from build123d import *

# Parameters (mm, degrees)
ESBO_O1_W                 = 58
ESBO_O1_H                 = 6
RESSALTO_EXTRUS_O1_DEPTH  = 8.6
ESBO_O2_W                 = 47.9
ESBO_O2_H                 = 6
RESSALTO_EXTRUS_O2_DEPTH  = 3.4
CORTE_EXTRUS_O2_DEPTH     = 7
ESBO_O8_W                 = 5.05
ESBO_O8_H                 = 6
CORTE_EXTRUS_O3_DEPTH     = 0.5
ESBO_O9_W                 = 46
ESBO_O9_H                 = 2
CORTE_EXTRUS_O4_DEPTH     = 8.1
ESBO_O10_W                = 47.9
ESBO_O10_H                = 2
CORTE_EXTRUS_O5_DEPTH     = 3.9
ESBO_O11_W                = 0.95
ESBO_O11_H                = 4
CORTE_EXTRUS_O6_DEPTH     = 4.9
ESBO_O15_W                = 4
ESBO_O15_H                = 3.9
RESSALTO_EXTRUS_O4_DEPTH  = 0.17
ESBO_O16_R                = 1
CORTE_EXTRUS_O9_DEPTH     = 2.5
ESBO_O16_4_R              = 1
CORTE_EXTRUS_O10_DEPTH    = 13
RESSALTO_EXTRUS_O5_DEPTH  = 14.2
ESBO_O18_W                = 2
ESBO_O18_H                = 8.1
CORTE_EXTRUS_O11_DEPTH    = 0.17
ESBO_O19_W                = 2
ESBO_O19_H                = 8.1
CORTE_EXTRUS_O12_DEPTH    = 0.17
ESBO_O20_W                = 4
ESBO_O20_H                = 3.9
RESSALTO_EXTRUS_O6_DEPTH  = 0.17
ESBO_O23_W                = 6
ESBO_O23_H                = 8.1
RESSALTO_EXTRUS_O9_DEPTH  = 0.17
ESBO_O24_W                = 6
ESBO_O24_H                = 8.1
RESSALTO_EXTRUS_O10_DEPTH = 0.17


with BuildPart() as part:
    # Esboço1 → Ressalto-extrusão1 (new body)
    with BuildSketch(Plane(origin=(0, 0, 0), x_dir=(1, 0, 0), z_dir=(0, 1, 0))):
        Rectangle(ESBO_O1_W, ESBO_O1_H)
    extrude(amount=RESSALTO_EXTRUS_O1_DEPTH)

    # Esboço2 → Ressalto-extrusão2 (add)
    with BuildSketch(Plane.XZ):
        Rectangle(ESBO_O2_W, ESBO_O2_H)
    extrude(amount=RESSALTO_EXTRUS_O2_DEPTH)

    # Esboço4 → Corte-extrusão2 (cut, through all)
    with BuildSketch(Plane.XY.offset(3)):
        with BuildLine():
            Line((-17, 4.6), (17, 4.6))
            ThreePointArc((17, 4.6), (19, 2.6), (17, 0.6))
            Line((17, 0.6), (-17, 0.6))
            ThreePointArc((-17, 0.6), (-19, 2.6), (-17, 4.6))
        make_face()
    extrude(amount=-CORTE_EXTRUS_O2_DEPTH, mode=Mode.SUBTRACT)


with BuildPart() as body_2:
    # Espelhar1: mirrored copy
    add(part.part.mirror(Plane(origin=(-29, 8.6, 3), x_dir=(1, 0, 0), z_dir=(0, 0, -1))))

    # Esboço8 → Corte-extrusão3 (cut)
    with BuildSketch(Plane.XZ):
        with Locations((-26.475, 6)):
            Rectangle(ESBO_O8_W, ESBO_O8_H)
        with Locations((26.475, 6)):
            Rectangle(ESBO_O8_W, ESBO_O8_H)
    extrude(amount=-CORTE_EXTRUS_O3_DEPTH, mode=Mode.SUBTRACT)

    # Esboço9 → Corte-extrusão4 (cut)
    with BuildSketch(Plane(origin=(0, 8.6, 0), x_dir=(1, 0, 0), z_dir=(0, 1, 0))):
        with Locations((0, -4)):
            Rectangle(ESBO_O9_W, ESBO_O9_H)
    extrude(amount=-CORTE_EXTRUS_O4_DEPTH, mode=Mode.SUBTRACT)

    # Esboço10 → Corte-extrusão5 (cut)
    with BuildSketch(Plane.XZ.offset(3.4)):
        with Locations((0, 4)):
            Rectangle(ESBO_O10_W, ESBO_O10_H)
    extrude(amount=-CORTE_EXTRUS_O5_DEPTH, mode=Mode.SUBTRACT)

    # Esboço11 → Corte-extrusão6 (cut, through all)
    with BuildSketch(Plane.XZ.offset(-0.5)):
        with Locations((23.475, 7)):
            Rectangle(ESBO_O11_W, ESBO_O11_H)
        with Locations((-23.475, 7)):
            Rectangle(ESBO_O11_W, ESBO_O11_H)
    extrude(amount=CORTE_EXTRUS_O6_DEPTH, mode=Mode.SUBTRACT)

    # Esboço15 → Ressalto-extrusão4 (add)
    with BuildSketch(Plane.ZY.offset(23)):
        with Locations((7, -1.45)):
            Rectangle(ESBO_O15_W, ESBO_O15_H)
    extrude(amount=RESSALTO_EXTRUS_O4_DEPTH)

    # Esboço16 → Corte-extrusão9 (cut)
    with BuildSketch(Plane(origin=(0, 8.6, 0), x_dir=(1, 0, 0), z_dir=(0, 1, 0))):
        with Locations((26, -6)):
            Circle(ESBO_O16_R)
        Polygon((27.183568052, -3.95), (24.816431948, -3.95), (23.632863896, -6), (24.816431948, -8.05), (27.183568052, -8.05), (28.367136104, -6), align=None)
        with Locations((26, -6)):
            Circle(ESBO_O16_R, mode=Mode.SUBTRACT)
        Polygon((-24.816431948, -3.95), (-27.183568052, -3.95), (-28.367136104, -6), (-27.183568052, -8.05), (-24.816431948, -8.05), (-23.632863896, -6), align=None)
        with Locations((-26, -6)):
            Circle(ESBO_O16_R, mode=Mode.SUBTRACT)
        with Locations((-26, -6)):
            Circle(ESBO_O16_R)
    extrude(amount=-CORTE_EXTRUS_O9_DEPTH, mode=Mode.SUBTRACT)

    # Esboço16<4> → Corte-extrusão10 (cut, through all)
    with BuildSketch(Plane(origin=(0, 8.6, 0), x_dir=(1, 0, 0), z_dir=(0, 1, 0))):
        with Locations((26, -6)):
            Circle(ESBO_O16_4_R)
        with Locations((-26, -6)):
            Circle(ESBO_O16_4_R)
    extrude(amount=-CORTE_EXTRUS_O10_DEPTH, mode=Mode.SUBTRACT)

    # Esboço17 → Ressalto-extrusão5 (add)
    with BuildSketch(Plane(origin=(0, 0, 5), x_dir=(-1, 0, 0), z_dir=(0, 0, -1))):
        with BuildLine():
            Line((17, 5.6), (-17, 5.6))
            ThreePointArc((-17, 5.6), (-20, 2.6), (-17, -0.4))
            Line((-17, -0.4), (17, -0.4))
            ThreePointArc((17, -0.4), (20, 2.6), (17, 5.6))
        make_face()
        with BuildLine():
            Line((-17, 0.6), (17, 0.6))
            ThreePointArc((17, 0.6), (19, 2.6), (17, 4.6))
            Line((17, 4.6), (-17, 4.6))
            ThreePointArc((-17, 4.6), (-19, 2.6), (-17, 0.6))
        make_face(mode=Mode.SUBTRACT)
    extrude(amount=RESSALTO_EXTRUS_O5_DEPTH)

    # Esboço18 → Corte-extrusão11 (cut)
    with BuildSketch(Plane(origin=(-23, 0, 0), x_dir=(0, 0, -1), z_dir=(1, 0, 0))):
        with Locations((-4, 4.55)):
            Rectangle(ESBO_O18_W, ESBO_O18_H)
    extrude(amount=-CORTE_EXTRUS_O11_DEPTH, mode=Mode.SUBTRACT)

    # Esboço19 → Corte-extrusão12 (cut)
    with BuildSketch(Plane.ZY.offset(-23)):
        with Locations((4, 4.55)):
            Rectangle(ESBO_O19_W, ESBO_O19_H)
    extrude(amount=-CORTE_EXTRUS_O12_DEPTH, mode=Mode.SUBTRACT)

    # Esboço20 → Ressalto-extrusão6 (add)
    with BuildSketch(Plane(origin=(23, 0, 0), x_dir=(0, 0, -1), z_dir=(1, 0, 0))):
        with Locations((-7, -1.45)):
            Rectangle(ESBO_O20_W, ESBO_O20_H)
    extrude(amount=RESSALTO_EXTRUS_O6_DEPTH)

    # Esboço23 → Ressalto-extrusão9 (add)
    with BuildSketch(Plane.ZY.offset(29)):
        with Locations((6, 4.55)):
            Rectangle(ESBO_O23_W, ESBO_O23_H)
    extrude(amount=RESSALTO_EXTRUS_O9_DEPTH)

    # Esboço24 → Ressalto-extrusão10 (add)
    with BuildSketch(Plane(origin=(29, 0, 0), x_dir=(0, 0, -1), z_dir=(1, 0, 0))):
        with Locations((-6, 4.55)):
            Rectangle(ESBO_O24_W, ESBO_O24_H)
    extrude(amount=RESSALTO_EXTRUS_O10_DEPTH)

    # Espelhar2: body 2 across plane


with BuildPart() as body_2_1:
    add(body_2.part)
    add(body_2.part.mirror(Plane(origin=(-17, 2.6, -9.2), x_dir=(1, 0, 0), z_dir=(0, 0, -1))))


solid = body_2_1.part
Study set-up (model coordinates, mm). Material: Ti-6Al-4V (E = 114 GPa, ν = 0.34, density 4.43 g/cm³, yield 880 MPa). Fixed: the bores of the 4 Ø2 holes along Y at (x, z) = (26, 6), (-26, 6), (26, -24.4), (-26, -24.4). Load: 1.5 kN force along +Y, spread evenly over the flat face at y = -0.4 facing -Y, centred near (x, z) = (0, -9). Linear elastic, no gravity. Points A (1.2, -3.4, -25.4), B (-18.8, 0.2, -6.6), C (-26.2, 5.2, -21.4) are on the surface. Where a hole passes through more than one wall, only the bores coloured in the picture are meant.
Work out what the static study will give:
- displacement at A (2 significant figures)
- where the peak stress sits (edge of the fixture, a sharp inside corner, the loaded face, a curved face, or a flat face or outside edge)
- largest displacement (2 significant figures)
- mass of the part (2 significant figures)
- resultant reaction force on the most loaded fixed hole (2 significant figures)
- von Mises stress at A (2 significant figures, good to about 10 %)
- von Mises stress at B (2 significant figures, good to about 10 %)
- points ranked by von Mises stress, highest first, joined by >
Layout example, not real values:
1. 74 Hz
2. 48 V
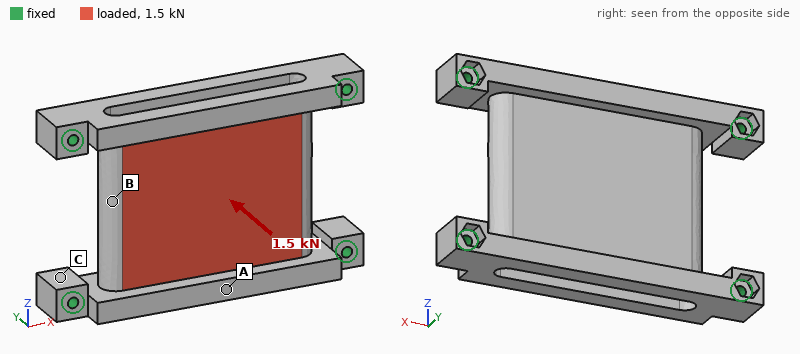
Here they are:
1. 0.069 mm
2. a curved face
3. 0.33 mm
4. 29 g
5. 460 N
6. 140 MPa
7. 250 MPa
8. B > A > C
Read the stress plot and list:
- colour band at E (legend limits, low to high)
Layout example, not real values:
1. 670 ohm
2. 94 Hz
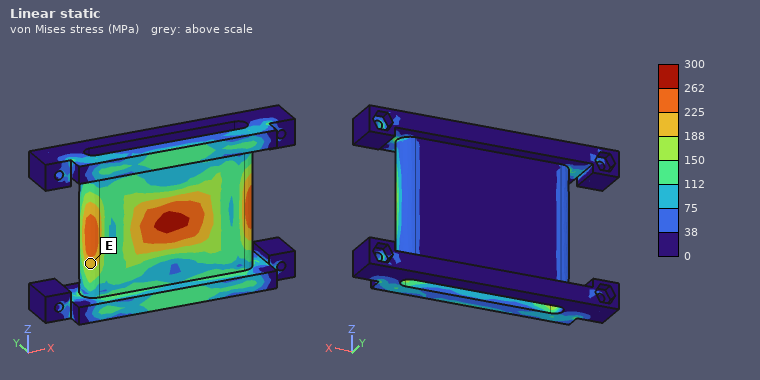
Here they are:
1. 188 to 225 MPa
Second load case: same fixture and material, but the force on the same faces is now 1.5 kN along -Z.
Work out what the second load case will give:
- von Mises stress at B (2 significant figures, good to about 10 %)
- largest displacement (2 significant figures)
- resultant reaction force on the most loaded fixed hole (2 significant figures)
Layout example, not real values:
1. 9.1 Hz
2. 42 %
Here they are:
1. 25 MPa
2. 18 µm
3. 390 N
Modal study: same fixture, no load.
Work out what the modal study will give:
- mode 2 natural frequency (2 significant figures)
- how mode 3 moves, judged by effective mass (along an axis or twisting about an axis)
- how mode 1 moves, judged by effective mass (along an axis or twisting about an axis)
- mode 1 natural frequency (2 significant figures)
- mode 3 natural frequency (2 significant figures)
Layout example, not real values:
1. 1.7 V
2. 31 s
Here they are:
1. 6500 Hz
2. twisting about X
3. along Y
4. 6100 Hz
5. 9400 Hz
